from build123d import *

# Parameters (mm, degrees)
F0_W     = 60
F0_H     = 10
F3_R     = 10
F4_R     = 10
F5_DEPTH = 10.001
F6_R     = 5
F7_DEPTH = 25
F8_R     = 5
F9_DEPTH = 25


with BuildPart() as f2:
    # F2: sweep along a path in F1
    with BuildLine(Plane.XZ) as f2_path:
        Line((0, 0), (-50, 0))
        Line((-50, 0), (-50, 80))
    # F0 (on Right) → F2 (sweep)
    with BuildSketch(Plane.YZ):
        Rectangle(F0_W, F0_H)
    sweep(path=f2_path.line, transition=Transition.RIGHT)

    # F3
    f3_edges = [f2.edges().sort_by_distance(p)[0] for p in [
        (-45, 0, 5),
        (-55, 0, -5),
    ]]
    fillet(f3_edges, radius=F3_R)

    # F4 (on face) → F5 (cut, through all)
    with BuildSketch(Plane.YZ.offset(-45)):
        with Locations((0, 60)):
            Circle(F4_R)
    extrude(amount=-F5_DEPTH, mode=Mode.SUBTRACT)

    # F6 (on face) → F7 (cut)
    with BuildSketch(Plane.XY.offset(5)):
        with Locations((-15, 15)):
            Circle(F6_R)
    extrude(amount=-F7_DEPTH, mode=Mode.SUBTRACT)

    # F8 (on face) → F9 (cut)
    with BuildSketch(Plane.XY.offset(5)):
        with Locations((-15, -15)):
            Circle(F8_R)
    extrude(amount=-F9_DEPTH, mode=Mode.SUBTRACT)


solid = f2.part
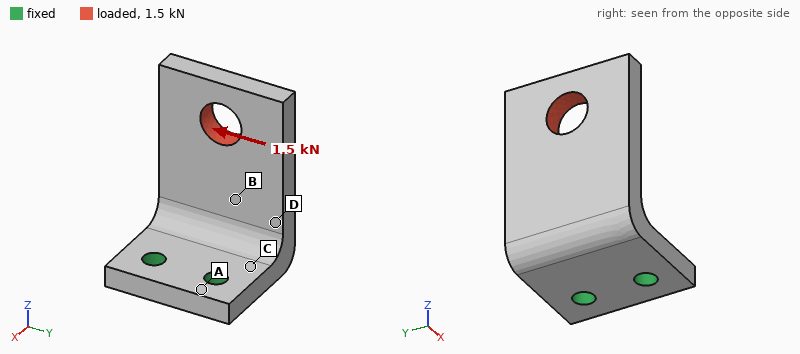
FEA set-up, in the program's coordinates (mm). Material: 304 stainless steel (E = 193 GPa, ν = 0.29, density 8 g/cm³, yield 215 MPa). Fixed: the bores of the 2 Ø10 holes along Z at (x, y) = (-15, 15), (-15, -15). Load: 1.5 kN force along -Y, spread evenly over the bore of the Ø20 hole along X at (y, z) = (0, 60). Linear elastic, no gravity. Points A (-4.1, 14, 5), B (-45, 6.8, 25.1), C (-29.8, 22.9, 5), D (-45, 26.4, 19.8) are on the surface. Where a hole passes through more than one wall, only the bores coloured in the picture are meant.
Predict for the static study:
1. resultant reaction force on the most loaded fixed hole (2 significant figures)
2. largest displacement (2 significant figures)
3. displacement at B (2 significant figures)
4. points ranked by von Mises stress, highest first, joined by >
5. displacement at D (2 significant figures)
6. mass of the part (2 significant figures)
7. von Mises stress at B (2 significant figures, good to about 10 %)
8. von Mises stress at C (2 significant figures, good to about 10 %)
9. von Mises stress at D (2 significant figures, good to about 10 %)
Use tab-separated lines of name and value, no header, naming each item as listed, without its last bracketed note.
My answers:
resultant reaction force on the most loaded fixed hole	2.7 kN
largest displacement	82 µm
displacement at B	25 µm
points ranked by von Mises stress, highest first, joined by >	C > D > B > A
displacement at D	30 µm
mass of the part	590 g
von Mises stress at B	14 MPa
von Mises stress at C	36 MPa
von Mises stress at D	24 MPa
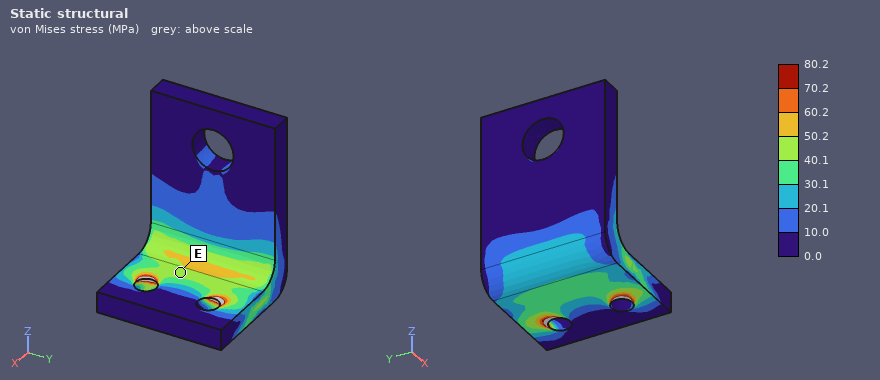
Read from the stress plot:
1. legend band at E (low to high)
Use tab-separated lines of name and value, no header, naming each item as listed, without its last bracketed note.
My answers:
legend band at E	40.1 to 50.2 MPa
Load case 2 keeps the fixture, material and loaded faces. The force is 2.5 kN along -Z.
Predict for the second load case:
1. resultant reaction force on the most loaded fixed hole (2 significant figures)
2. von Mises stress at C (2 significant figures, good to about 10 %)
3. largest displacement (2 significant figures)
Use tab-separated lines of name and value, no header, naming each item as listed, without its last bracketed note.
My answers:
resultant reaction force on the most loaded fixed hole	1.3 kN
von Mises stress at C	47 MPa
largest displacement	0.11 mm
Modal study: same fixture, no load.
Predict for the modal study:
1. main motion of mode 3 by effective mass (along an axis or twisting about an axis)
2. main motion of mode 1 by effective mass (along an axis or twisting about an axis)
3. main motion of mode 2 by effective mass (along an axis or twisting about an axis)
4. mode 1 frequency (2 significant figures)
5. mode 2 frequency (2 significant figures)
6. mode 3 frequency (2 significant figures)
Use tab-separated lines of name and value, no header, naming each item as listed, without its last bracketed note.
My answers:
main motion of mode 3 by effective mass	along Z
main motion of mode 1 by effective mass	along X
main motion of mode 2 by effective mass	along Y
mode 1 frequency	890 Hz
mode 2 frequency	1700 Hz
mode 3 frequency	3200 Hz
